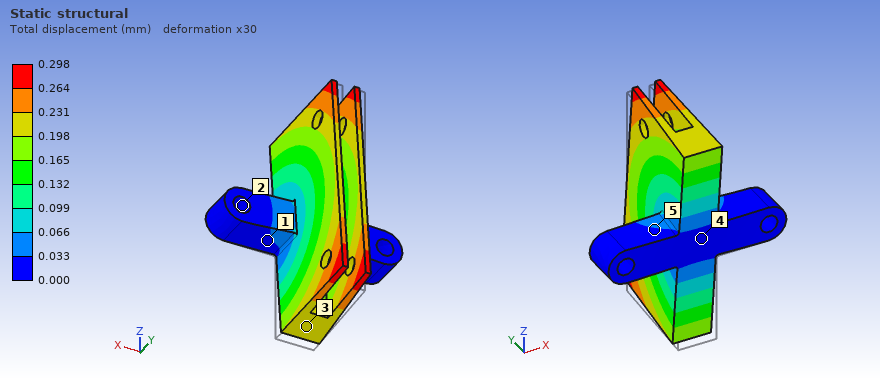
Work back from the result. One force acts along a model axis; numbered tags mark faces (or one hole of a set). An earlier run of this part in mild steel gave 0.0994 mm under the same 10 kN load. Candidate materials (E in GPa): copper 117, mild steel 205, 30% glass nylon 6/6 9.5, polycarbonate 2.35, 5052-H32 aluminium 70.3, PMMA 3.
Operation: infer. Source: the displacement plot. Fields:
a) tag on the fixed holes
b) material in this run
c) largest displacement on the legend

2
5052-H32 aluminium
0.298 mm
